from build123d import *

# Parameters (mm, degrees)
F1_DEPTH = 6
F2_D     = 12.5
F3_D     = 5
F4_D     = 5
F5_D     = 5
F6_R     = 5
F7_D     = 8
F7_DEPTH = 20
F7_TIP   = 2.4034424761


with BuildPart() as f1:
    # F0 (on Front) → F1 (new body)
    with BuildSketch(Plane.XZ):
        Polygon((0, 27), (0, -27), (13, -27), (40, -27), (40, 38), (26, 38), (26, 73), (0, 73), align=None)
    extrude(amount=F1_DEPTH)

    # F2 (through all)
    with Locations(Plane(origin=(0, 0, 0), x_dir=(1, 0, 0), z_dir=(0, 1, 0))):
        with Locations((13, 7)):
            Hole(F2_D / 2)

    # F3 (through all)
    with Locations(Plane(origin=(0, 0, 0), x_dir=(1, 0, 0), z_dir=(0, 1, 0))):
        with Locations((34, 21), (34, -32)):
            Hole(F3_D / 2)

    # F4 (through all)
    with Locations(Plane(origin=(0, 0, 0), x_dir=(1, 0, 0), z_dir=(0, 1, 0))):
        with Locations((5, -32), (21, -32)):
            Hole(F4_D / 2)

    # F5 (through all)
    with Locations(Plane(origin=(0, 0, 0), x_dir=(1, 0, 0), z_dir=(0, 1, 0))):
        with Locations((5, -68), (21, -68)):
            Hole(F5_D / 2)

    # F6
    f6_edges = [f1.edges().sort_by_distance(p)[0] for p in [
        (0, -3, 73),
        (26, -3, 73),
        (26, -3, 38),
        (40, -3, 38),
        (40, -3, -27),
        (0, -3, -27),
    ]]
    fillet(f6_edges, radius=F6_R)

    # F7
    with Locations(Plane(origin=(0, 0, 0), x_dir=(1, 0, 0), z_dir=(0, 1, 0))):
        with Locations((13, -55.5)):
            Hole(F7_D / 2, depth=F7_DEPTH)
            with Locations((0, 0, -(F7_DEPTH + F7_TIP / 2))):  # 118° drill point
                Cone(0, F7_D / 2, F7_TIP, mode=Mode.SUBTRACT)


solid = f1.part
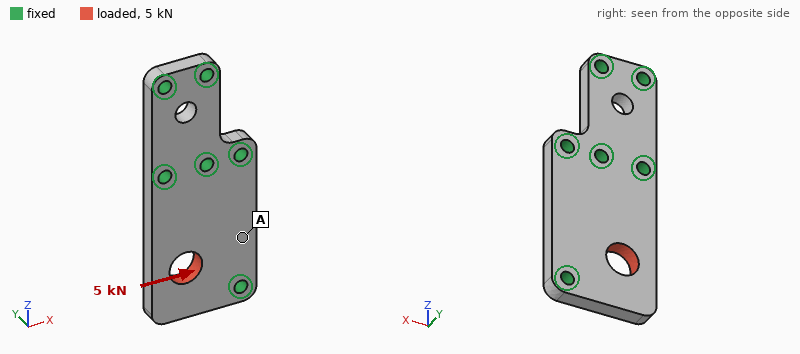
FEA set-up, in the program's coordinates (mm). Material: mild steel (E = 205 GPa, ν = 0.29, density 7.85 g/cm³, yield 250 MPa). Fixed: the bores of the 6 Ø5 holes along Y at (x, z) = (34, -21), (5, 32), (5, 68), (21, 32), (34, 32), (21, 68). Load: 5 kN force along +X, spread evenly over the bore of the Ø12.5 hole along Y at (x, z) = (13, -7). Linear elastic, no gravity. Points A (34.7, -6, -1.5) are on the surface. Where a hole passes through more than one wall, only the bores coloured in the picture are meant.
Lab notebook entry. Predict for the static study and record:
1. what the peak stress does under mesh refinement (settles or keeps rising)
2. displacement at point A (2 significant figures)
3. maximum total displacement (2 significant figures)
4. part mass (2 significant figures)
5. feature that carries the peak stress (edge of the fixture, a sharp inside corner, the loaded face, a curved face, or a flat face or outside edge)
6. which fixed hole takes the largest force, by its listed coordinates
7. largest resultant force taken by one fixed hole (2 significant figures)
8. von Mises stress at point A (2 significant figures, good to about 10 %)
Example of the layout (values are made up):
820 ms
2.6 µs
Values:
keeps rising
3.6 µm
6.7 µm
150 g
edge of the fixture
(34, -21)
3.3 kN
9.6 MPa
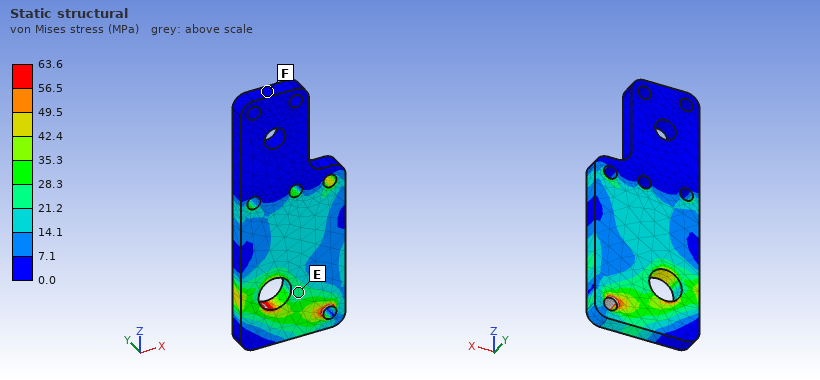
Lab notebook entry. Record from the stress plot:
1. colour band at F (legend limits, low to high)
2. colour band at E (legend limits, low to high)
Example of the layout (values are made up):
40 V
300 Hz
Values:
0.0 to 7.1 MPa
21.2 to 28.3 MPa
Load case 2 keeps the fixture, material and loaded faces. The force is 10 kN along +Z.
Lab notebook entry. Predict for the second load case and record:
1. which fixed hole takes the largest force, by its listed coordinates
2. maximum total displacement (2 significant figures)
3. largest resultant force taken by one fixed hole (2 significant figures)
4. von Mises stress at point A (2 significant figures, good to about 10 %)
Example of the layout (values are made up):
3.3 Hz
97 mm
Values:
(34, -21)
12 µm
3.5 kN
13 MPa
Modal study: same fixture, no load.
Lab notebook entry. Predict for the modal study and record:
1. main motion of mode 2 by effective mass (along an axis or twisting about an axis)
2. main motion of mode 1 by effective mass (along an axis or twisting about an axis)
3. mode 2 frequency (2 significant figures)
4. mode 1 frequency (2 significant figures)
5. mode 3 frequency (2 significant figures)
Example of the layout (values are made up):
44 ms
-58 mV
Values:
along Y
along Y
10 kHz
5300 Hz
14 kHz
